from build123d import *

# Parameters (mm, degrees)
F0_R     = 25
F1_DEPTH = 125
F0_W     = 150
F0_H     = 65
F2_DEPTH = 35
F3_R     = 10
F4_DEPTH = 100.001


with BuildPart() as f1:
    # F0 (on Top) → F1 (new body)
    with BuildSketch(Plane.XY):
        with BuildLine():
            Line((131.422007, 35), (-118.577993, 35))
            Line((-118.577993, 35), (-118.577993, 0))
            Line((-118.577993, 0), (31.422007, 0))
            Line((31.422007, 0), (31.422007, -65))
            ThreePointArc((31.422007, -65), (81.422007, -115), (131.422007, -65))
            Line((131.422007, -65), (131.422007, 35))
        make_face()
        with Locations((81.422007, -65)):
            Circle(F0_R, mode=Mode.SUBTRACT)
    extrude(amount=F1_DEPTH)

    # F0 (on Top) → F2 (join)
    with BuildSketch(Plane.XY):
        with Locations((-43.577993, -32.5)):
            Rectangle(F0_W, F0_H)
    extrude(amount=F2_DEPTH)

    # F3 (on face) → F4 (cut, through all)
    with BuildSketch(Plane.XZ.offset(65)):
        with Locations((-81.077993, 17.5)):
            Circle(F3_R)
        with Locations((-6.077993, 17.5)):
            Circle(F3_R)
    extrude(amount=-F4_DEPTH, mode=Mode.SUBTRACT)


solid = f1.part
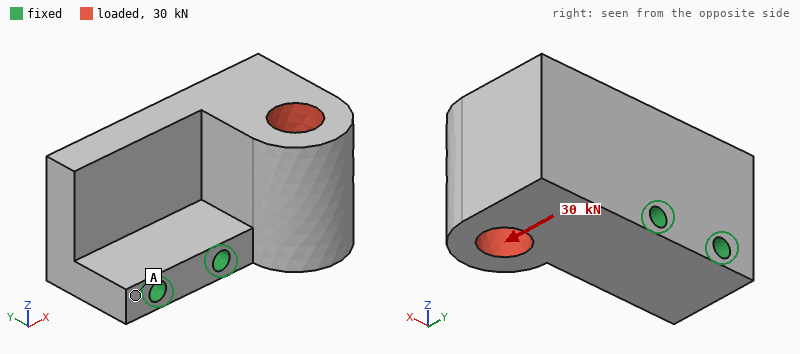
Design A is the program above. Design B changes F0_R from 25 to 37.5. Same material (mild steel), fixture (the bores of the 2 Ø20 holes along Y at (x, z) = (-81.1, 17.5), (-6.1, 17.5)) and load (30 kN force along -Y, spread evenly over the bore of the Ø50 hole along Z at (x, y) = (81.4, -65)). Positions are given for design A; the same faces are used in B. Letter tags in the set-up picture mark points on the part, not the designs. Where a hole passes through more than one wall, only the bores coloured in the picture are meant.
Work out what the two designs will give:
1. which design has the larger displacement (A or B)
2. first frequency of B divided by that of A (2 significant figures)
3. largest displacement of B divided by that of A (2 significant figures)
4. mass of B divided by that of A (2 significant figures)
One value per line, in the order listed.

B
1.1
1.3
0.87
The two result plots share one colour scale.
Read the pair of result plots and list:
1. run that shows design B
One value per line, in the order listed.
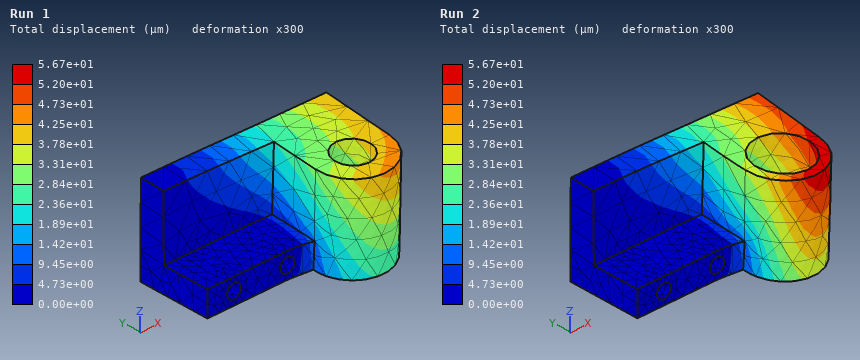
Run 2
